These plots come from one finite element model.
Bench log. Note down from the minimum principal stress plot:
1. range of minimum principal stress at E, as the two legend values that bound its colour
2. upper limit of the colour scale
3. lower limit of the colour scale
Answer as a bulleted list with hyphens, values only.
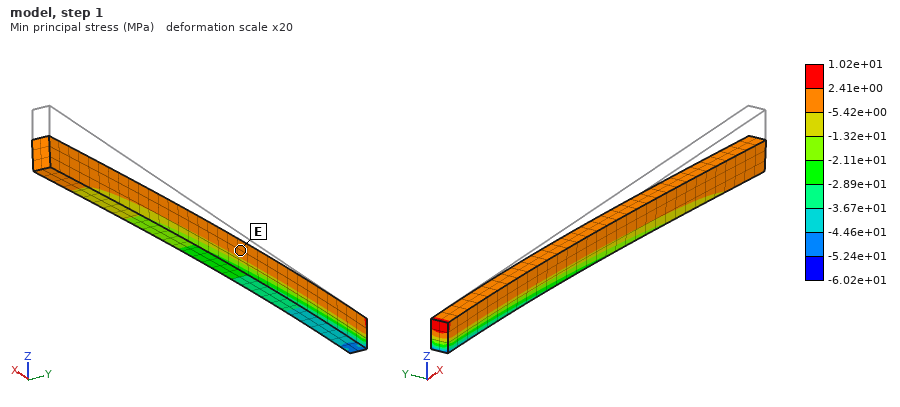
- -5.42e+00 to 2.41e+00 MPa
- 1.02e+01 MPa
- -6.02e+01 MPa
